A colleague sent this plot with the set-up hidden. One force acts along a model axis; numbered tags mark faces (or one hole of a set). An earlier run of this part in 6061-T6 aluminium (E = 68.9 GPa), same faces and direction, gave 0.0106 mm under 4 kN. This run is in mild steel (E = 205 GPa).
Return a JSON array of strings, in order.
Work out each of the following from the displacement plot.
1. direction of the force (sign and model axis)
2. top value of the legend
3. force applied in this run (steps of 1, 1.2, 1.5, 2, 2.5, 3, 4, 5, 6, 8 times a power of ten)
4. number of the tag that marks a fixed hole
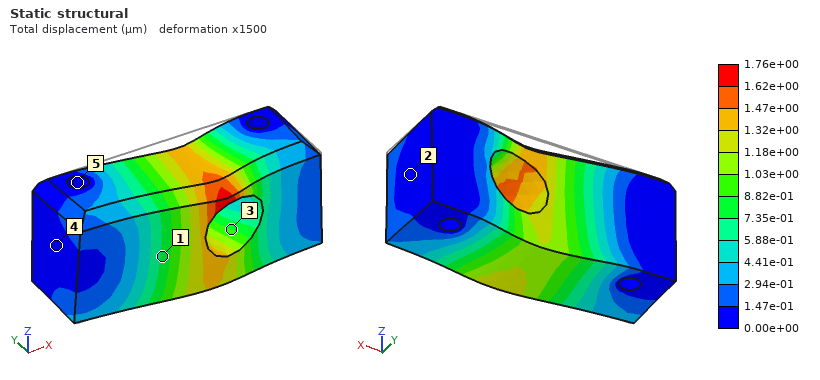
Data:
["-Z", "1.76e+00 µm", "2 kN", "5"]
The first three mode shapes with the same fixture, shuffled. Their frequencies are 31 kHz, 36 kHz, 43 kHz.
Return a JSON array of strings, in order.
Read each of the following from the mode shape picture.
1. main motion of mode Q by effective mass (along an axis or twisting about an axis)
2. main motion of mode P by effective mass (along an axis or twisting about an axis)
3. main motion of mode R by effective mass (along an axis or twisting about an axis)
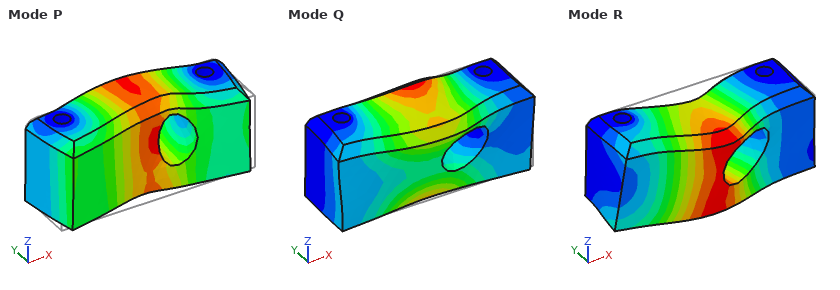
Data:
["twisting about X", "along Y", "along Z"]
